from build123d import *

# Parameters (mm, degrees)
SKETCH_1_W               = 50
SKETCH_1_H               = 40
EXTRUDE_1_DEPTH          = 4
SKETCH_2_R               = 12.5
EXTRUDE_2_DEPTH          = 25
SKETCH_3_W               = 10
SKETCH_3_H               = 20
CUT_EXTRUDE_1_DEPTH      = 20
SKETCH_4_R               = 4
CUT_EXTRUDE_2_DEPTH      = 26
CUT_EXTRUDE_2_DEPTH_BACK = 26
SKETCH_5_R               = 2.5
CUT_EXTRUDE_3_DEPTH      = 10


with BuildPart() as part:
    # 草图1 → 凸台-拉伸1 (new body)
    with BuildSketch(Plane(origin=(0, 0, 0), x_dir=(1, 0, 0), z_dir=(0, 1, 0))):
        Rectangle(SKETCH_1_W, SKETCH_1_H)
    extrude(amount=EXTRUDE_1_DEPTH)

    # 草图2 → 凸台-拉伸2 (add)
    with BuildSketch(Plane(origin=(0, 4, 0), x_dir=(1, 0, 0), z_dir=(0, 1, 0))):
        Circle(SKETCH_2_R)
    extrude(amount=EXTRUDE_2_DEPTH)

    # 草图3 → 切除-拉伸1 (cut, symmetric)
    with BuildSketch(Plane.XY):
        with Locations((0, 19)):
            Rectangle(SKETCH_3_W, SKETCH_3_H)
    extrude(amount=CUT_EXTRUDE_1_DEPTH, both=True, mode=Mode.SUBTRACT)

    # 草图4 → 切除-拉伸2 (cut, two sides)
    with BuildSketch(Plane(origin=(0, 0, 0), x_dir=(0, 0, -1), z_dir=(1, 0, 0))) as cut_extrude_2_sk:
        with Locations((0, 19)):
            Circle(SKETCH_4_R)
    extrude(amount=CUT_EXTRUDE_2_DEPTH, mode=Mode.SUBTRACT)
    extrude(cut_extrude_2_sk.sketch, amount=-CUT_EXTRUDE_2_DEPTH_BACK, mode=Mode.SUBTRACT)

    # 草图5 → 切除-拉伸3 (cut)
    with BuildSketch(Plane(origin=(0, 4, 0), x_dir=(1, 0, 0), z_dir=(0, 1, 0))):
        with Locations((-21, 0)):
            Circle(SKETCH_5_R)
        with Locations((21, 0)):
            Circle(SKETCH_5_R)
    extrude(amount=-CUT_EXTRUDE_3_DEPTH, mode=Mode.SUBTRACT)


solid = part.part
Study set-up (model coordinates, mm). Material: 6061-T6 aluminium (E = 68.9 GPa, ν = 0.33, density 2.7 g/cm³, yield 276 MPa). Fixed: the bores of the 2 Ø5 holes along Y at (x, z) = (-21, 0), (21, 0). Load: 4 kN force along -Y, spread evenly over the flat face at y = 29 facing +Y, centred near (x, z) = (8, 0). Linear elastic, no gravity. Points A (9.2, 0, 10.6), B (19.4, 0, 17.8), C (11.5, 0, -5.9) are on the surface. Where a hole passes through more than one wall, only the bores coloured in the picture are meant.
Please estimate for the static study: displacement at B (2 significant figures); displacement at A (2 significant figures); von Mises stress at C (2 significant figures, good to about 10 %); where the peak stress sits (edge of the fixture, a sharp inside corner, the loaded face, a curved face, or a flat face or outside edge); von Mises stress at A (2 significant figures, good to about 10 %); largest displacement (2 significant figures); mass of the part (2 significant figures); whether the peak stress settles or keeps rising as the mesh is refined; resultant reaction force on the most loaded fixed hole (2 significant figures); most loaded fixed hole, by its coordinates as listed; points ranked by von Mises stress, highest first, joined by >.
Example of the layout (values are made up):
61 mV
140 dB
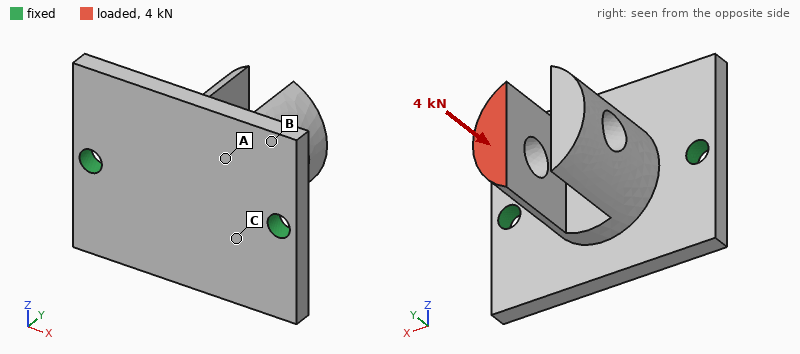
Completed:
33 µm
53 µm
100 MPa
edge of the fixture
67 MPa
80 µm
39 g
keeps rising
3.1 kN
(21, 0)
C > A > B
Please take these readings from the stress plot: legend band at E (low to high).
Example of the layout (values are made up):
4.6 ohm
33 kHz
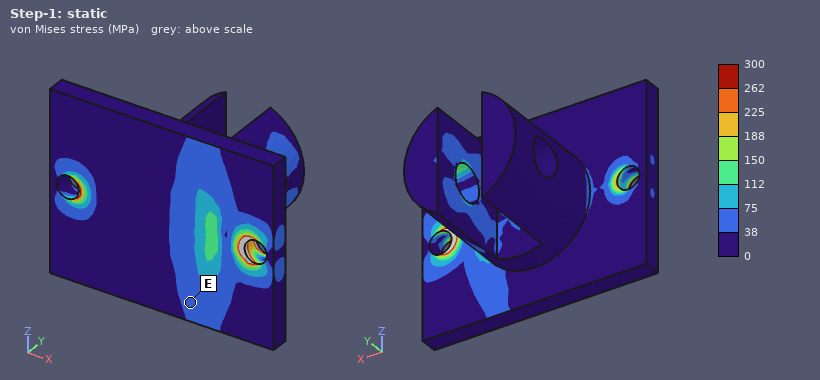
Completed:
38 to 75 MPa
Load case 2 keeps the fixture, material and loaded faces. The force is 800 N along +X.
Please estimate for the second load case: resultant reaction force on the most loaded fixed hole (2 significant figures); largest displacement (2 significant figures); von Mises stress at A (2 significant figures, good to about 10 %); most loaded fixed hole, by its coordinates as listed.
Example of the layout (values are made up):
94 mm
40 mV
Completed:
990 N
0.18 mm
13 MPa
(-21, 0)
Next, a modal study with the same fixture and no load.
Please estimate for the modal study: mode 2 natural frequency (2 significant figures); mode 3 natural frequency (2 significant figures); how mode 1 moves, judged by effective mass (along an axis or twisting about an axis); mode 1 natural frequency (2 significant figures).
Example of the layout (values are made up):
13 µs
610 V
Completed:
7400 Hz
7700 Hz
along Z
3500 Hz
